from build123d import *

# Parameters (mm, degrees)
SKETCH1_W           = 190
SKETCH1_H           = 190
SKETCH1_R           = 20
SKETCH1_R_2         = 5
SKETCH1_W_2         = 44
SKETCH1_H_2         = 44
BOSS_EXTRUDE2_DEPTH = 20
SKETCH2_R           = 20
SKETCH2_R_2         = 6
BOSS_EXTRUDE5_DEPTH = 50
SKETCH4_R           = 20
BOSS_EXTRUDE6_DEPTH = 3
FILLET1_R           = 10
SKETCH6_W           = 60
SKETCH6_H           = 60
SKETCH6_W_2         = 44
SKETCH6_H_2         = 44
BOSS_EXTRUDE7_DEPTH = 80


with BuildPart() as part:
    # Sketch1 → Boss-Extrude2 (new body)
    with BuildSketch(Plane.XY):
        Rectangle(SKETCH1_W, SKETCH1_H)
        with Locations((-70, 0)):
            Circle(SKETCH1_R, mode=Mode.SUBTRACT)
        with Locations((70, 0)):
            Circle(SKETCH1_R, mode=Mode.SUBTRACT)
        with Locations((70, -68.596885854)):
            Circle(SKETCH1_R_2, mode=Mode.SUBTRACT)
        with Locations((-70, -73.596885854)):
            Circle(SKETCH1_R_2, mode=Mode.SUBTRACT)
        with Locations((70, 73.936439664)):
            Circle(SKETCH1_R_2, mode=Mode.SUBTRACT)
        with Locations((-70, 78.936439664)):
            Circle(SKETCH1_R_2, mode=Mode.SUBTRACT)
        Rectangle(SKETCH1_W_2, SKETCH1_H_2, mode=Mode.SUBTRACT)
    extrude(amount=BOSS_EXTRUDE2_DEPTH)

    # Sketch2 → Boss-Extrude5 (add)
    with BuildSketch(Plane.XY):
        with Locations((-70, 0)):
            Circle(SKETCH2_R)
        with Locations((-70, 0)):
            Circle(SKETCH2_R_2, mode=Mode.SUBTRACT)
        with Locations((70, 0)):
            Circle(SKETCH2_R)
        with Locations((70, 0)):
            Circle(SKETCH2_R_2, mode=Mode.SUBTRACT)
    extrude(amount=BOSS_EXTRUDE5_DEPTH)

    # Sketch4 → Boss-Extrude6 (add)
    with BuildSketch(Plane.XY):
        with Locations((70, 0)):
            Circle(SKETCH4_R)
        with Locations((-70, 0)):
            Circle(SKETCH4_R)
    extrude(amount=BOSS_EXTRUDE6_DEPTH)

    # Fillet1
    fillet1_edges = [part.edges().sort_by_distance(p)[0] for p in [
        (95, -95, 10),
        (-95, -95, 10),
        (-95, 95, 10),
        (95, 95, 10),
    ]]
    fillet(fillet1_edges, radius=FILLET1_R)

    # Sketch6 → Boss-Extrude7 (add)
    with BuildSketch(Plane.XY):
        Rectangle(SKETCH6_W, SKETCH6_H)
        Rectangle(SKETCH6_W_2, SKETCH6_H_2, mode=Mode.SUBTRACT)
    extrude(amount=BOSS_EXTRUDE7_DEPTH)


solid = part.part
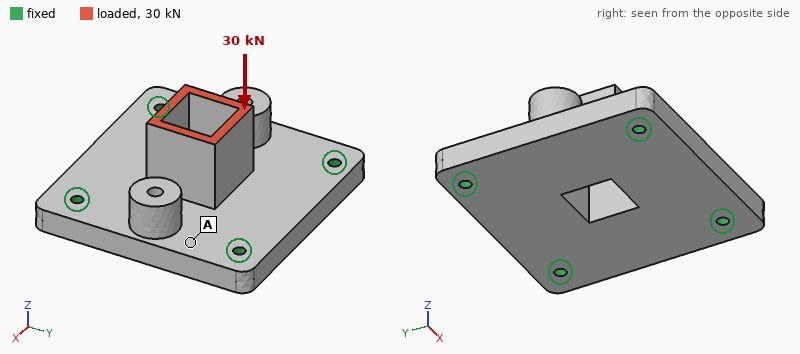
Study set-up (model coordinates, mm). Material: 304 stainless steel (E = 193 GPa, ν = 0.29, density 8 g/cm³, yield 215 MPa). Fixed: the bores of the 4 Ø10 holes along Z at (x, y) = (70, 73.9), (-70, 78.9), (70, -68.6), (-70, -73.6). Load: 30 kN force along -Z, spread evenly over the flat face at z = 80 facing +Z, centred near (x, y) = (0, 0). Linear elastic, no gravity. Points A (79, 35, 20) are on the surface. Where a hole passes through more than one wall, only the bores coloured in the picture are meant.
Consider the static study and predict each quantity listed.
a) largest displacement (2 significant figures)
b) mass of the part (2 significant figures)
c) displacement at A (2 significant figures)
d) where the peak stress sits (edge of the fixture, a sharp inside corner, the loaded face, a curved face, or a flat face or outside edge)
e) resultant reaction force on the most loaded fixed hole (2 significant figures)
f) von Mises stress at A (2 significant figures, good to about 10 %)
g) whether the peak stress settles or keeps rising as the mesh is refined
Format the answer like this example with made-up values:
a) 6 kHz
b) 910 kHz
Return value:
a) 54 µm
b) 6.7 kg
c) 11 µm
d) edge of the fixture
e) 8.3 kN
f) 18 MPa
g) keeps rising
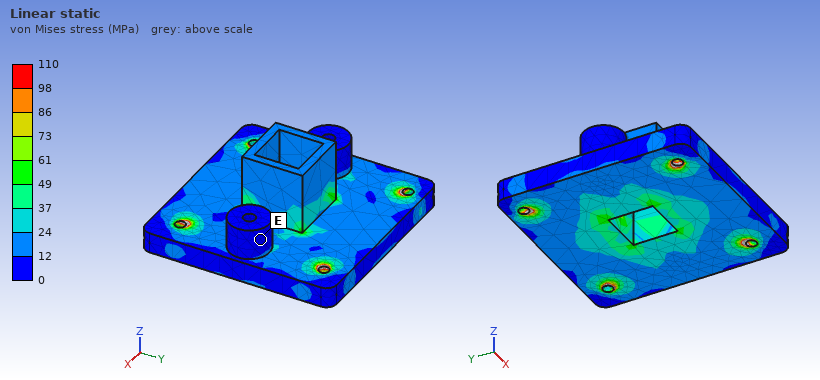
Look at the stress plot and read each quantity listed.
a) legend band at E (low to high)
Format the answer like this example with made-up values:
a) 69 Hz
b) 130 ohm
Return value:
a) 0 to 12 MPa
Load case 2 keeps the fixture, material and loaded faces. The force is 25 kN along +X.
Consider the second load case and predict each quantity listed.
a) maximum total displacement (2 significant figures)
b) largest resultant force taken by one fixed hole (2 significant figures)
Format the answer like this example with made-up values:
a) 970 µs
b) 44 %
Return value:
a) 0.14 mm
b) 11 kN
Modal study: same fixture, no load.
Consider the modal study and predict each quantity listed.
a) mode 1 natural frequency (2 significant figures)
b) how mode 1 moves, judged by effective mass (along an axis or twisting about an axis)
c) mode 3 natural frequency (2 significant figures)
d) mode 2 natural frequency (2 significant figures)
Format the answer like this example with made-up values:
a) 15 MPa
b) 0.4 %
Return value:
a) 2500 Hz
b) along Z
c) 3600 Hz
d) 3200 Hz
